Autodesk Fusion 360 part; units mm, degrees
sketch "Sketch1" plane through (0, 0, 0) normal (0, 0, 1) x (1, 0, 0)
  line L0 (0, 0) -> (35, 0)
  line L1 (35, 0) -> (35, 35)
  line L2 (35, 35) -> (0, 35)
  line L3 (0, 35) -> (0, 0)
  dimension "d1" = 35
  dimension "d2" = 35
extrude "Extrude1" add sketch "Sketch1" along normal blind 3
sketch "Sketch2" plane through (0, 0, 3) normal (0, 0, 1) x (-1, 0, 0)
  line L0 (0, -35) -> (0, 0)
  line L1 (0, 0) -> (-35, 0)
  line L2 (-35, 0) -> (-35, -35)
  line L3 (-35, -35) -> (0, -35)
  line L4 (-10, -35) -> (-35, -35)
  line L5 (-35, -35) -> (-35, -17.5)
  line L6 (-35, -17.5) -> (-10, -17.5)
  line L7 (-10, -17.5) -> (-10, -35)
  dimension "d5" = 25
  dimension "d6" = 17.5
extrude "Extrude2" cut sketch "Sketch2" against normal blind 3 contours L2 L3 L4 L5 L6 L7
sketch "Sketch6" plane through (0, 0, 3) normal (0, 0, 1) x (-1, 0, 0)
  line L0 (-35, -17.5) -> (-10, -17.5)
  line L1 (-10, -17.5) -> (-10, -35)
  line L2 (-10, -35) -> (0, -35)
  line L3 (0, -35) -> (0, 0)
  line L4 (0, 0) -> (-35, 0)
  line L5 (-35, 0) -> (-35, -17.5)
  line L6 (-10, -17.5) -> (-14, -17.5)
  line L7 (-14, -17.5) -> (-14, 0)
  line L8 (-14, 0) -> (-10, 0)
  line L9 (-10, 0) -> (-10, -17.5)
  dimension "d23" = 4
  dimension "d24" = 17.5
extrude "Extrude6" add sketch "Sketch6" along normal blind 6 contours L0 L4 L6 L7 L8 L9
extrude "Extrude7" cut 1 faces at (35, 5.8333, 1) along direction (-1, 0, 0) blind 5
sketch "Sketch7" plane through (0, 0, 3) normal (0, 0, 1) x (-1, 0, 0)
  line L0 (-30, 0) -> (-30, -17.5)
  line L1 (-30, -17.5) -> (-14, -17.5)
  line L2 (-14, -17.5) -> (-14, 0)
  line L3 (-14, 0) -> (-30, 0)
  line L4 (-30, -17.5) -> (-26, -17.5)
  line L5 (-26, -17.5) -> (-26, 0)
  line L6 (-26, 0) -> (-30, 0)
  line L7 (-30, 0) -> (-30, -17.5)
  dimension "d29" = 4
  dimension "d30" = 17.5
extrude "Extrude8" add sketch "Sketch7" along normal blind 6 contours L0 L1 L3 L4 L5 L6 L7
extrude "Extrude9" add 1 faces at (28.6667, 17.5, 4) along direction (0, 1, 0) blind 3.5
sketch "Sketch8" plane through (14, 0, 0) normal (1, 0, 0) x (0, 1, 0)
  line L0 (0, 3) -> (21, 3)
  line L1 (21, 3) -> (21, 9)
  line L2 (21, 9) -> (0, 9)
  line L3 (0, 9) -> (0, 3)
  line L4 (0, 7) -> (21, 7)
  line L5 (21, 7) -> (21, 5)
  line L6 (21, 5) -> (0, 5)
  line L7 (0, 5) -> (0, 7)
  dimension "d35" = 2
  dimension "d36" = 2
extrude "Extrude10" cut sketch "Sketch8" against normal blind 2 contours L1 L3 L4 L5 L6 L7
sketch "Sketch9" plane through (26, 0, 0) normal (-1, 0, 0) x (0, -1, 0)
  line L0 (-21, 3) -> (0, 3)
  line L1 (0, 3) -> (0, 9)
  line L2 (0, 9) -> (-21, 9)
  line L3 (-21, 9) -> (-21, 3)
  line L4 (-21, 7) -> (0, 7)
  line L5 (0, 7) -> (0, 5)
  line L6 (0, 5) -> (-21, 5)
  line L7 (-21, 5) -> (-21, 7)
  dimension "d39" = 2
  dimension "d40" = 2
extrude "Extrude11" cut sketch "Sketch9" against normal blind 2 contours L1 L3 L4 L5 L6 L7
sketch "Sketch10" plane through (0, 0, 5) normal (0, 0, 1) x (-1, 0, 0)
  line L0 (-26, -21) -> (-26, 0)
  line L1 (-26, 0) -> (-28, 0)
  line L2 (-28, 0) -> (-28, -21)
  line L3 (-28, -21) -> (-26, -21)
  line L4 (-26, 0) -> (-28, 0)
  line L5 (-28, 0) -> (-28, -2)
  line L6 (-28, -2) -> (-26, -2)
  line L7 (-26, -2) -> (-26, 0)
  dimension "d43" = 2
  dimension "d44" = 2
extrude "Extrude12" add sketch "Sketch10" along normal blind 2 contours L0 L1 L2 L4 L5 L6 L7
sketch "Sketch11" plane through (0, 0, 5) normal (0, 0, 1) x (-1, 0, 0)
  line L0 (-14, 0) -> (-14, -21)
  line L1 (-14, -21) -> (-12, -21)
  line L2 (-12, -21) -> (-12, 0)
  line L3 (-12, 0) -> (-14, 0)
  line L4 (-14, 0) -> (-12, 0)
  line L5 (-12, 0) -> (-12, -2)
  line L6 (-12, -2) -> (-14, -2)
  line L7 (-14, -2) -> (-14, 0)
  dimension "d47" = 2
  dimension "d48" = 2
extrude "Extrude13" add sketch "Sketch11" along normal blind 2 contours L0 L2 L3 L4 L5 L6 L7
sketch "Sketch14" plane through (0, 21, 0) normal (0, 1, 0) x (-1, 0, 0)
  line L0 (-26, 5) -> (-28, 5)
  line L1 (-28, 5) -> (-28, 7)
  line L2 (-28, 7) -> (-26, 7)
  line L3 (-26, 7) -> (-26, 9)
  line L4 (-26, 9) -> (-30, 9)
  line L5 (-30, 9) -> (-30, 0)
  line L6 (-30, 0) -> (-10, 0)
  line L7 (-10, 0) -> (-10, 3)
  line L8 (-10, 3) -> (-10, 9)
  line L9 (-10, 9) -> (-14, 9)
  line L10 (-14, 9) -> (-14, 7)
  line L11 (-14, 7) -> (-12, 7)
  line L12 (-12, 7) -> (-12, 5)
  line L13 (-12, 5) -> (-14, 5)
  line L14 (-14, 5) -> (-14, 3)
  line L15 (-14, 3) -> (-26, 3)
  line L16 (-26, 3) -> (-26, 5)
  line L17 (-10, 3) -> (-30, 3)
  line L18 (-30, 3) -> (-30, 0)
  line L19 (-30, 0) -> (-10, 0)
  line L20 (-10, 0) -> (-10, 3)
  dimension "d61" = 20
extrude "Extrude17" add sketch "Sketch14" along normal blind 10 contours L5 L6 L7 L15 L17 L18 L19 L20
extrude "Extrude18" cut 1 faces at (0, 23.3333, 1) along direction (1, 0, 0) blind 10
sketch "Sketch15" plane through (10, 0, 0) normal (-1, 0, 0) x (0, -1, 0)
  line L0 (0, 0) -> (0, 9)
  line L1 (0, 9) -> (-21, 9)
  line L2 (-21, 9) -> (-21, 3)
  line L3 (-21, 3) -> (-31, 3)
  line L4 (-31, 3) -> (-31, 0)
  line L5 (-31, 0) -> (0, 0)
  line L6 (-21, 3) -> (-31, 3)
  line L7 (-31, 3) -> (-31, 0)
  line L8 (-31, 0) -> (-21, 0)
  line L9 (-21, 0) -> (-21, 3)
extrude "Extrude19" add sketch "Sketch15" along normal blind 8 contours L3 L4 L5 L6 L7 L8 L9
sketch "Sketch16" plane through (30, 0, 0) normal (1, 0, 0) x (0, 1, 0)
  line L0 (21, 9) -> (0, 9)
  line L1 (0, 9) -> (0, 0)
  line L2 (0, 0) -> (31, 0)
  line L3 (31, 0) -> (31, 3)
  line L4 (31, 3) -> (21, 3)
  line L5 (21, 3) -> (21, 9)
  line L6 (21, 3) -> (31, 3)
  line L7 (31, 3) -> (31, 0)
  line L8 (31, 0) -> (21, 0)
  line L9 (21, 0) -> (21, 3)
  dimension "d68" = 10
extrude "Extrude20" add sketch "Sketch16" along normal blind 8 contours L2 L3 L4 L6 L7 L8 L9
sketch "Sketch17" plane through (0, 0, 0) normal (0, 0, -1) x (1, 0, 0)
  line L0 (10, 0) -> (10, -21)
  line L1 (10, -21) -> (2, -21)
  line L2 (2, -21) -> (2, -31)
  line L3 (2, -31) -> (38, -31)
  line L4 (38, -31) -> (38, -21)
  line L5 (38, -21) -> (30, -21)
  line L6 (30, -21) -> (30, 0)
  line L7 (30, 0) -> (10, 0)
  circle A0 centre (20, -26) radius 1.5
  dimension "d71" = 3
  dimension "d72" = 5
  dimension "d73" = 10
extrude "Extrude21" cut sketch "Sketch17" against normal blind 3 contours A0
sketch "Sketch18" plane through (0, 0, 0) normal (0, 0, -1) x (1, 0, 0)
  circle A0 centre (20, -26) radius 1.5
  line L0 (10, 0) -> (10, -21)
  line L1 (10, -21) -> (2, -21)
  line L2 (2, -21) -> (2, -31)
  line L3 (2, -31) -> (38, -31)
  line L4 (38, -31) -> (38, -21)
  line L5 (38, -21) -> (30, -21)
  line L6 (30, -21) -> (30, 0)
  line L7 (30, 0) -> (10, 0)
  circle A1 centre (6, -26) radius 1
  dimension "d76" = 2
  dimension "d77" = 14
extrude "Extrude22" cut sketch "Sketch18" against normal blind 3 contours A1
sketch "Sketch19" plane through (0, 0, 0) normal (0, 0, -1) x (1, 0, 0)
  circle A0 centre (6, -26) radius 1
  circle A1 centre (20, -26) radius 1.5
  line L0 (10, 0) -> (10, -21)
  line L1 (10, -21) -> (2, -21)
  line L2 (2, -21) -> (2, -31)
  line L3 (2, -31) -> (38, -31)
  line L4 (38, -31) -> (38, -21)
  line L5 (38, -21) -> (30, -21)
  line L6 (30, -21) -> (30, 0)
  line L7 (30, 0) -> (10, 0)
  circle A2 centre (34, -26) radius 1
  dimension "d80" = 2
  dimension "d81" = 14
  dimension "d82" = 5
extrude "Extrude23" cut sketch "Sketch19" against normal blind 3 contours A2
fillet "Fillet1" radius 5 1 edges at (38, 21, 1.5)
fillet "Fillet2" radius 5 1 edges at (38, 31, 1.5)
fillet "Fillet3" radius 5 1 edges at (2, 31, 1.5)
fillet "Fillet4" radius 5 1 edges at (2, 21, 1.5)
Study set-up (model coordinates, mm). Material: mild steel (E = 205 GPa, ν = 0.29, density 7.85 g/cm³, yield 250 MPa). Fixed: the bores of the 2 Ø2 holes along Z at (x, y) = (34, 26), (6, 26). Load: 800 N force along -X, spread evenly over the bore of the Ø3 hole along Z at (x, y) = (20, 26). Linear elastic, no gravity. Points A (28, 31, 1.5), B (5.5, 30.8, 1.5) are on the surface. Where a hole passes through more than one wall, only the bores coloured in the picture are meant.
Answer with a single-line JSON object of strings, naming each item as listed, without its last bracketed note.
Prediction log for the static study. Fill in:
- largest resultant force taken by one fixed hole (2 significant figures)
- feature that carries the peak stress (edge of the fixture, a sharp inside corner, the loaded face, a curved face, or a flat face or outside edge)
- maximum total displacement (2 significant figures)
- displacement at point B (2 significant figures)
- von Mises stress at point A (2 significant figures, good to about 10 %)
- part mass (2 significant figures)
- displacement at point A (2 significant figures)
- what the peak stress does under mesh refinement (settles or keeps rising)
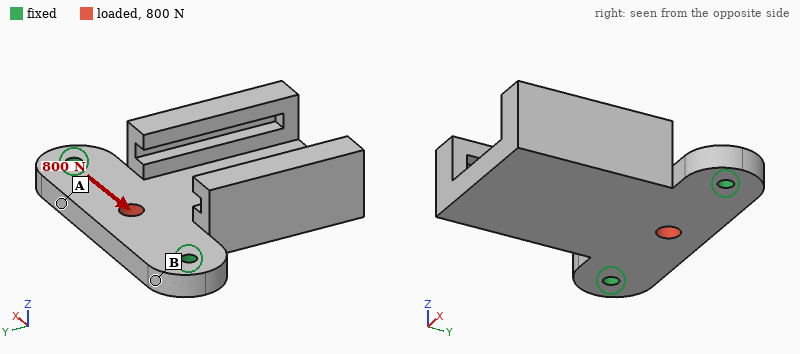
{"largest resultant force taken by one fixed hole": "400 N", "feature that carries the peak stress": "edge of the fixture", "maximum total displacement": "1.2 µm", "displacement at point B": "0.33 µm", "von Mises stress at point A": "11 MPa", "part mass": "24 g", "displacement at point A": "0.57 µm", "what the peak stress does under mesh refinement": "keeps rising"}
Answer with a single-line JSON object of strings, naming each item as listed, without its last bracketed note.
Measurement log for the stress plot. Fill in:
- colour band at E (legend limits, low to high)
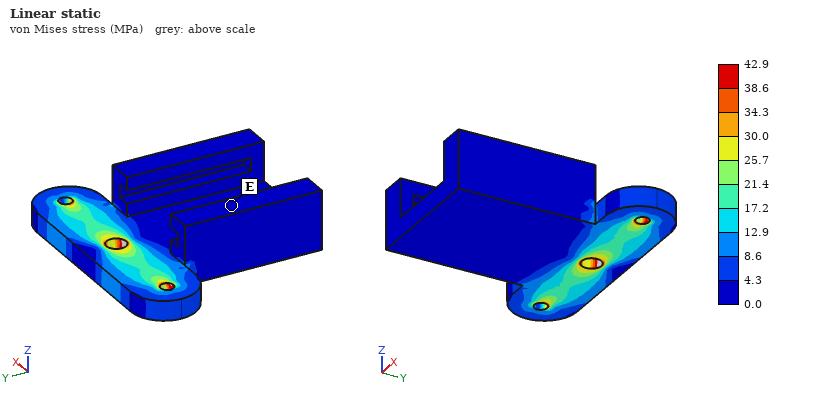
{"colour band at E": "0.0 to 4.3 MPa"}
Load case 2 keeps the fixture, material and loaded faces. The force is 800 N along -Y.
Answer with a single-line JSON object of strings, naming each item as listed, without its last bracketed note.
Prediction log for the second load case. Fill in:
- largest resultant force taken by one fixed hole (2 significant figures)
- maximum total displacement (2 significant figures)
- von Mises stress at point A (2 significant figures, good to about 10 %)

{"largest resultant force taken by one fixed hole": "420 N", "maximum total displacement": "4.0 µm", "von Mises stress at point A": "14 MPa"}
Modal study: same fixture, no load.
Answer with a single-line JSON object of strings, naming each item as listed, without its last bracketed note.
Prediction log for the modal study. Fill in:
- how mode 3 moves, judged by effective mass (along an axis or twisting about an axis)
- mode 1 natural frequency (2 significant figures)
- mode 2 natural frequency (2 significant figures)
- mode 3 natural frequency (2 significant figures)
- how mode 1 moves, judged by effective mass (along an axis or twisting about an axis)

{"how mode 3 moves, judged by effective mass": "along X", "mode 1 natural frequency": "2400 Hz", "mode 2 natural frequency": "7600 Hz", "mode 3 natural frequency": "13 kHz", "how mode 1 moves, judged by effective mass": "along Z"}
